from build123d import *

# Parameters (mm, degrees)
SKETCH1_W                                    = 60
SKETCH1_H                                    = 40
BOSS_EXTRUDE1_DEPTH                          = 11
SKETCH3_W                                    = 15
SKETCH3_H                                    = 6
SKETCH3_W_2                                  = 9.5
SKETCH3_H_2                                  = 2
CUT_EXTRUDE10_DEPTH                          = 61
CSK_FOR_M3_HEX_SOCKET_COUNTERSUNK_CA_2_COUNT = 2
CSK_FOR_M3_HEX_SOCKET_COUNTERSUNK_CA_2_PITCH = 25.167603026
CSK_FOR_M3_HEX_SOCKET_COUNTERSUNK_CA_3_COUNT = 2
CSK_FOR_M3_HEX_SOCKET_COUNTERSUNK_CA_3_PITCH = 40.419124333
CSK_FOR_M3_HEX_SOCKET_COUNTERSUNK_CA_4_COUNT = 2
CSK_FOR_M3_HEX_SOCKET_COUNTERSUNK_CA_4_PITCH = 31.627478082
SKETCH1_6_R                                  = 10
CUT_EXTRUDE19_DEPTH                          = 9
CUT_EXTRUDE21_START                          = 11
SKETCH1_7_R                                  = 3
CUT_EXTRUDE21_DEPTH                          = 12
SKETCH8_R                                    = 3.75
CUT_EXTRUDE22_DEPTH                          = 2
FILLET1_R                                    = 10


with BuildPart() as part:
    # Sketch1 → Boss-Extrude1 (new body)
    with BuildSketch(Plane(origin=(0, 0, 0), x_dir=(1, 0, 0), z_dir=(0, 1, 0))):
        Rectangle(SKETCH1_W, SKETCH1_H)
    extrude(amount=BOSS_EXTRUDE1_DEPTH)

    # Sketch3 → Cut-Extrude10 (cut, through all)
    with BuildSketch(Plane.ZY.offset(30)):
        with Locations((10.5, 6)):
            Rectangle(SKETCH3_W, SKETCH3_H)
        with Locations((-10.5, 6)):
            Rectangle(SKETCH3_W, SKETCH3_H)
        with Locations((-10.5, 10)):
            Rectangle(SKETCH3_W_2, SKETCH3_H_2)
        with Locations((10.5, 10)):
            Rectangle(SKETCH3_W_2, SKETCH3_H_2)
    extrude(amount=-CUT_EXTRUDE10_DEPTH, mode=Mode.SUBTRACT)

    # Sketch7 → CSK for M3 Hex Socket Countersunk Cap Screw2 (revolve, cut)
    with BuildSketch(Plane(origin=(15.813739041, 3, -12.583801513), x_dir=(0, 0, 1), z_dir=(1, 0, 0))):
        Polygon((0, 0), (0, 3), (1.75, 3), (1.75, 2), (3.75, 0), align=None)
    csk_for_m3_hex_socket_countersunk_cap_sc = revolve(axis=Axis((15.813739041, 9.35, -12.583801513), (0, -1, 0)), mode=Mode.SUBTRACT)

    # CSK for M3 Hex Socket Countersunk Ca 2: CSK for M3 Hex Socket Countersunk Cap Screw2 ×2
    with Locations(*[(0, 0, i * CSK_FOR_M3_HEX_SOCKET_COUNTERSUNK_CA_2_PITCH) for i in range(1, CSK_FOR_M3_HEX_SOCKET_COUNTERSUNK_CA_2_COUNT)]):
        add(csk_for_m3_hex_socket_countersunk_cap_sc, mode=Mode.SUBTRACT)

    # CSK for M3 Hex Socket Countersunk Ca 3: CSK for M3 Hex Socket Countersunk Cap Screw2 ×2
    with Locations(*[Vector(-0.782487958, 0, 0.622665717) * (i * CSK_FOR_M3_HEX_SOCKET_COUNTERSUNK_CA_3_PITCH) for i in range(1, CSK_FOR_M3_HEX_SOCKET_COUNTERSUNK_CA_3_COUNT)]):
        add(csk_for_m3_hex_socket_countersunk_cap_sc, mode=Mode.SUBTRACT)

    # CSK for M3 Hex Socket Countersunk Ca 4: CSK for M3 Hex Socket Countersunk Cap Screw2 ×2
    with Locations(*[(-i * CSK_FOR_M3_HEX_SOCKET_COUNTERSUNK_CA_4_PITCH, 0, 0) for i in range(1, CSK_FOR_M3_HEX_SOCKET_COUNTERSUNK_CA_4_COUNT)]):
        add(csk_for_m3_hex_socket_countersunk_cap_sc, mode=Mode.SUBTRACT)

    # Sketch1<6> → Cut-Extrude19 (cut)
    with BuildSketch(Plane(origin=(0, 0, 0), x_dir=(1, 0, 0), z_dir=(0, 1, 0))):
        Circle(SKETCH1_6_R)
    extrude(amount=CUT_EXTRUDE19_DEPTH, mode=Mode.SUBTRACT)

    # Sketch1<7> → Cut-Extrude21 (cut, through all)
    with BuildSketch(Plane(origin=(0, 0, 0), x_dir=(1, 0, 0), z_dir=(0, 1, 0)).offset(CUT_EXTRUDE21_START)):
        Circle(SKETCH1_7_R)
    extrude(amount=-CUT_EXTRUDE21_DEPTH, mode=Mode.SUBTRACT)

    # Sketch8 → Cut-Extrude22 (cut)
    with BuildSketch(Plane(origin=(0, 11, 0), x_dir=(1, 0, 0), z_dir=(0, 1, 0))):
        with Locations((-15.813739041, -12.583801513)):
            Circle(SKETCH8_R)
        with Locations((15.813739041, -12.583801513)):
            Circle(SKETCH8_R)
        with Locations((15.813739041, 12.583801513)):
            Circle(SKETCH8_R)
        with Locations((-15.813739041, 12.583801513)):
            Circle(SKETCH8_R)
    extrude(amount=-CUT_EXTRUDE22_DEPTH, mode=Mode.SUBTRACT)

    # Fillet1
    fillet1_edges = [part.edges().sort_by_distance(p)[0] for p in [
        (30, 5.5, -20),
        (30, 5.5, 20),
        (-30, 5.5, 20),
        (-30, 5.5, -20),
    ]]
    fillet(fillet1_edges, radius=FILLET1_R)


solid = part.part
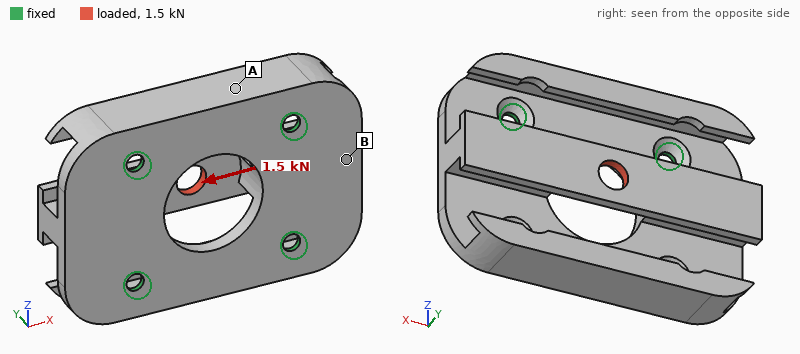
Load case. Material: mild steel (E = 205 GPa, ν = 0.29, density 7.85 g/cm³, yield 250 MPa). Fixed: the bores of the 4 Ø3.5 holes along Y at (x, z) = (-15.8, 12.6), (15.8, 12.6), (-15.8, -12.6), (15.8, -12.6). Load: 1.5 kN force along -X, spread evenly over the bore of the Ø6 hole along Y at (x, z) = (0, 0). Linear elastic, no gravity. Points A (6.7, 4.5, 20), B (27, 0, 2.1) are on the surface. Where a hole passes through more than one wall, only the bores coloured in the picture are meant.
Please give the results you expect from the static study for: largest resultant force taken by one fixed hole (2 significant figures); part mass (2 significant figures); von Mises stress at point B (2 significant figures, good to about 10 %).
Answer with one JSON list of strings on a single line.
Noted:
["420 N", "84 g", "49 MPa"]
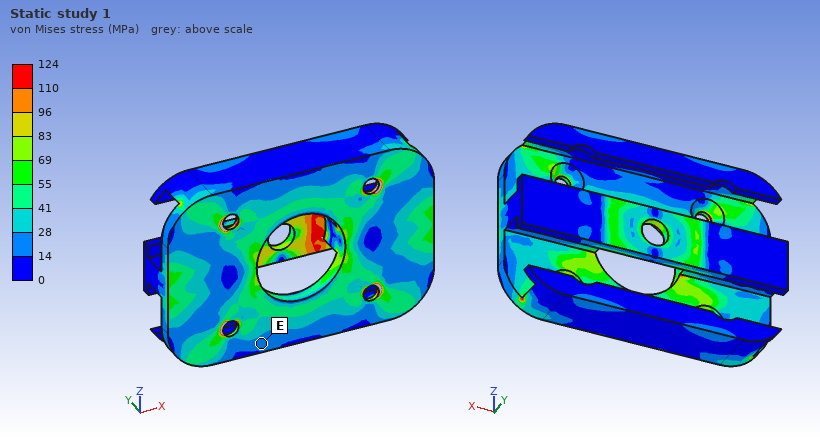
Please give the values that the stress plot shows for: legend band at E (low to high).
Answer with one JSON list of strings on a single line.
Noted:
["14 to 28 MPa"]
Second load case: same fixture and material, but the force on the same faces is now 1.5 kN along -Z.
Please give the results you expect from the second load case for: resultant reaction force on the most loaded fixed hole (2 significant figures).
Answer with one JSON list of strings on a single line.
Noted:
["510 N"]
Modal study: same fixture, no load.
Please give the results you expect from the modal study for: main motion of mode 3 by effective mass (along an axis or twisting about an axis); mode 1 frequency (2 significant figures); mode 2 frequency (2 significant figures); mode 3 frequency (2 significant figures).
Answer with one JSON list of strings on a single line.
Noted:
["along Z", "7200 Hz", "7600 Hz", "8100 Hz"]
